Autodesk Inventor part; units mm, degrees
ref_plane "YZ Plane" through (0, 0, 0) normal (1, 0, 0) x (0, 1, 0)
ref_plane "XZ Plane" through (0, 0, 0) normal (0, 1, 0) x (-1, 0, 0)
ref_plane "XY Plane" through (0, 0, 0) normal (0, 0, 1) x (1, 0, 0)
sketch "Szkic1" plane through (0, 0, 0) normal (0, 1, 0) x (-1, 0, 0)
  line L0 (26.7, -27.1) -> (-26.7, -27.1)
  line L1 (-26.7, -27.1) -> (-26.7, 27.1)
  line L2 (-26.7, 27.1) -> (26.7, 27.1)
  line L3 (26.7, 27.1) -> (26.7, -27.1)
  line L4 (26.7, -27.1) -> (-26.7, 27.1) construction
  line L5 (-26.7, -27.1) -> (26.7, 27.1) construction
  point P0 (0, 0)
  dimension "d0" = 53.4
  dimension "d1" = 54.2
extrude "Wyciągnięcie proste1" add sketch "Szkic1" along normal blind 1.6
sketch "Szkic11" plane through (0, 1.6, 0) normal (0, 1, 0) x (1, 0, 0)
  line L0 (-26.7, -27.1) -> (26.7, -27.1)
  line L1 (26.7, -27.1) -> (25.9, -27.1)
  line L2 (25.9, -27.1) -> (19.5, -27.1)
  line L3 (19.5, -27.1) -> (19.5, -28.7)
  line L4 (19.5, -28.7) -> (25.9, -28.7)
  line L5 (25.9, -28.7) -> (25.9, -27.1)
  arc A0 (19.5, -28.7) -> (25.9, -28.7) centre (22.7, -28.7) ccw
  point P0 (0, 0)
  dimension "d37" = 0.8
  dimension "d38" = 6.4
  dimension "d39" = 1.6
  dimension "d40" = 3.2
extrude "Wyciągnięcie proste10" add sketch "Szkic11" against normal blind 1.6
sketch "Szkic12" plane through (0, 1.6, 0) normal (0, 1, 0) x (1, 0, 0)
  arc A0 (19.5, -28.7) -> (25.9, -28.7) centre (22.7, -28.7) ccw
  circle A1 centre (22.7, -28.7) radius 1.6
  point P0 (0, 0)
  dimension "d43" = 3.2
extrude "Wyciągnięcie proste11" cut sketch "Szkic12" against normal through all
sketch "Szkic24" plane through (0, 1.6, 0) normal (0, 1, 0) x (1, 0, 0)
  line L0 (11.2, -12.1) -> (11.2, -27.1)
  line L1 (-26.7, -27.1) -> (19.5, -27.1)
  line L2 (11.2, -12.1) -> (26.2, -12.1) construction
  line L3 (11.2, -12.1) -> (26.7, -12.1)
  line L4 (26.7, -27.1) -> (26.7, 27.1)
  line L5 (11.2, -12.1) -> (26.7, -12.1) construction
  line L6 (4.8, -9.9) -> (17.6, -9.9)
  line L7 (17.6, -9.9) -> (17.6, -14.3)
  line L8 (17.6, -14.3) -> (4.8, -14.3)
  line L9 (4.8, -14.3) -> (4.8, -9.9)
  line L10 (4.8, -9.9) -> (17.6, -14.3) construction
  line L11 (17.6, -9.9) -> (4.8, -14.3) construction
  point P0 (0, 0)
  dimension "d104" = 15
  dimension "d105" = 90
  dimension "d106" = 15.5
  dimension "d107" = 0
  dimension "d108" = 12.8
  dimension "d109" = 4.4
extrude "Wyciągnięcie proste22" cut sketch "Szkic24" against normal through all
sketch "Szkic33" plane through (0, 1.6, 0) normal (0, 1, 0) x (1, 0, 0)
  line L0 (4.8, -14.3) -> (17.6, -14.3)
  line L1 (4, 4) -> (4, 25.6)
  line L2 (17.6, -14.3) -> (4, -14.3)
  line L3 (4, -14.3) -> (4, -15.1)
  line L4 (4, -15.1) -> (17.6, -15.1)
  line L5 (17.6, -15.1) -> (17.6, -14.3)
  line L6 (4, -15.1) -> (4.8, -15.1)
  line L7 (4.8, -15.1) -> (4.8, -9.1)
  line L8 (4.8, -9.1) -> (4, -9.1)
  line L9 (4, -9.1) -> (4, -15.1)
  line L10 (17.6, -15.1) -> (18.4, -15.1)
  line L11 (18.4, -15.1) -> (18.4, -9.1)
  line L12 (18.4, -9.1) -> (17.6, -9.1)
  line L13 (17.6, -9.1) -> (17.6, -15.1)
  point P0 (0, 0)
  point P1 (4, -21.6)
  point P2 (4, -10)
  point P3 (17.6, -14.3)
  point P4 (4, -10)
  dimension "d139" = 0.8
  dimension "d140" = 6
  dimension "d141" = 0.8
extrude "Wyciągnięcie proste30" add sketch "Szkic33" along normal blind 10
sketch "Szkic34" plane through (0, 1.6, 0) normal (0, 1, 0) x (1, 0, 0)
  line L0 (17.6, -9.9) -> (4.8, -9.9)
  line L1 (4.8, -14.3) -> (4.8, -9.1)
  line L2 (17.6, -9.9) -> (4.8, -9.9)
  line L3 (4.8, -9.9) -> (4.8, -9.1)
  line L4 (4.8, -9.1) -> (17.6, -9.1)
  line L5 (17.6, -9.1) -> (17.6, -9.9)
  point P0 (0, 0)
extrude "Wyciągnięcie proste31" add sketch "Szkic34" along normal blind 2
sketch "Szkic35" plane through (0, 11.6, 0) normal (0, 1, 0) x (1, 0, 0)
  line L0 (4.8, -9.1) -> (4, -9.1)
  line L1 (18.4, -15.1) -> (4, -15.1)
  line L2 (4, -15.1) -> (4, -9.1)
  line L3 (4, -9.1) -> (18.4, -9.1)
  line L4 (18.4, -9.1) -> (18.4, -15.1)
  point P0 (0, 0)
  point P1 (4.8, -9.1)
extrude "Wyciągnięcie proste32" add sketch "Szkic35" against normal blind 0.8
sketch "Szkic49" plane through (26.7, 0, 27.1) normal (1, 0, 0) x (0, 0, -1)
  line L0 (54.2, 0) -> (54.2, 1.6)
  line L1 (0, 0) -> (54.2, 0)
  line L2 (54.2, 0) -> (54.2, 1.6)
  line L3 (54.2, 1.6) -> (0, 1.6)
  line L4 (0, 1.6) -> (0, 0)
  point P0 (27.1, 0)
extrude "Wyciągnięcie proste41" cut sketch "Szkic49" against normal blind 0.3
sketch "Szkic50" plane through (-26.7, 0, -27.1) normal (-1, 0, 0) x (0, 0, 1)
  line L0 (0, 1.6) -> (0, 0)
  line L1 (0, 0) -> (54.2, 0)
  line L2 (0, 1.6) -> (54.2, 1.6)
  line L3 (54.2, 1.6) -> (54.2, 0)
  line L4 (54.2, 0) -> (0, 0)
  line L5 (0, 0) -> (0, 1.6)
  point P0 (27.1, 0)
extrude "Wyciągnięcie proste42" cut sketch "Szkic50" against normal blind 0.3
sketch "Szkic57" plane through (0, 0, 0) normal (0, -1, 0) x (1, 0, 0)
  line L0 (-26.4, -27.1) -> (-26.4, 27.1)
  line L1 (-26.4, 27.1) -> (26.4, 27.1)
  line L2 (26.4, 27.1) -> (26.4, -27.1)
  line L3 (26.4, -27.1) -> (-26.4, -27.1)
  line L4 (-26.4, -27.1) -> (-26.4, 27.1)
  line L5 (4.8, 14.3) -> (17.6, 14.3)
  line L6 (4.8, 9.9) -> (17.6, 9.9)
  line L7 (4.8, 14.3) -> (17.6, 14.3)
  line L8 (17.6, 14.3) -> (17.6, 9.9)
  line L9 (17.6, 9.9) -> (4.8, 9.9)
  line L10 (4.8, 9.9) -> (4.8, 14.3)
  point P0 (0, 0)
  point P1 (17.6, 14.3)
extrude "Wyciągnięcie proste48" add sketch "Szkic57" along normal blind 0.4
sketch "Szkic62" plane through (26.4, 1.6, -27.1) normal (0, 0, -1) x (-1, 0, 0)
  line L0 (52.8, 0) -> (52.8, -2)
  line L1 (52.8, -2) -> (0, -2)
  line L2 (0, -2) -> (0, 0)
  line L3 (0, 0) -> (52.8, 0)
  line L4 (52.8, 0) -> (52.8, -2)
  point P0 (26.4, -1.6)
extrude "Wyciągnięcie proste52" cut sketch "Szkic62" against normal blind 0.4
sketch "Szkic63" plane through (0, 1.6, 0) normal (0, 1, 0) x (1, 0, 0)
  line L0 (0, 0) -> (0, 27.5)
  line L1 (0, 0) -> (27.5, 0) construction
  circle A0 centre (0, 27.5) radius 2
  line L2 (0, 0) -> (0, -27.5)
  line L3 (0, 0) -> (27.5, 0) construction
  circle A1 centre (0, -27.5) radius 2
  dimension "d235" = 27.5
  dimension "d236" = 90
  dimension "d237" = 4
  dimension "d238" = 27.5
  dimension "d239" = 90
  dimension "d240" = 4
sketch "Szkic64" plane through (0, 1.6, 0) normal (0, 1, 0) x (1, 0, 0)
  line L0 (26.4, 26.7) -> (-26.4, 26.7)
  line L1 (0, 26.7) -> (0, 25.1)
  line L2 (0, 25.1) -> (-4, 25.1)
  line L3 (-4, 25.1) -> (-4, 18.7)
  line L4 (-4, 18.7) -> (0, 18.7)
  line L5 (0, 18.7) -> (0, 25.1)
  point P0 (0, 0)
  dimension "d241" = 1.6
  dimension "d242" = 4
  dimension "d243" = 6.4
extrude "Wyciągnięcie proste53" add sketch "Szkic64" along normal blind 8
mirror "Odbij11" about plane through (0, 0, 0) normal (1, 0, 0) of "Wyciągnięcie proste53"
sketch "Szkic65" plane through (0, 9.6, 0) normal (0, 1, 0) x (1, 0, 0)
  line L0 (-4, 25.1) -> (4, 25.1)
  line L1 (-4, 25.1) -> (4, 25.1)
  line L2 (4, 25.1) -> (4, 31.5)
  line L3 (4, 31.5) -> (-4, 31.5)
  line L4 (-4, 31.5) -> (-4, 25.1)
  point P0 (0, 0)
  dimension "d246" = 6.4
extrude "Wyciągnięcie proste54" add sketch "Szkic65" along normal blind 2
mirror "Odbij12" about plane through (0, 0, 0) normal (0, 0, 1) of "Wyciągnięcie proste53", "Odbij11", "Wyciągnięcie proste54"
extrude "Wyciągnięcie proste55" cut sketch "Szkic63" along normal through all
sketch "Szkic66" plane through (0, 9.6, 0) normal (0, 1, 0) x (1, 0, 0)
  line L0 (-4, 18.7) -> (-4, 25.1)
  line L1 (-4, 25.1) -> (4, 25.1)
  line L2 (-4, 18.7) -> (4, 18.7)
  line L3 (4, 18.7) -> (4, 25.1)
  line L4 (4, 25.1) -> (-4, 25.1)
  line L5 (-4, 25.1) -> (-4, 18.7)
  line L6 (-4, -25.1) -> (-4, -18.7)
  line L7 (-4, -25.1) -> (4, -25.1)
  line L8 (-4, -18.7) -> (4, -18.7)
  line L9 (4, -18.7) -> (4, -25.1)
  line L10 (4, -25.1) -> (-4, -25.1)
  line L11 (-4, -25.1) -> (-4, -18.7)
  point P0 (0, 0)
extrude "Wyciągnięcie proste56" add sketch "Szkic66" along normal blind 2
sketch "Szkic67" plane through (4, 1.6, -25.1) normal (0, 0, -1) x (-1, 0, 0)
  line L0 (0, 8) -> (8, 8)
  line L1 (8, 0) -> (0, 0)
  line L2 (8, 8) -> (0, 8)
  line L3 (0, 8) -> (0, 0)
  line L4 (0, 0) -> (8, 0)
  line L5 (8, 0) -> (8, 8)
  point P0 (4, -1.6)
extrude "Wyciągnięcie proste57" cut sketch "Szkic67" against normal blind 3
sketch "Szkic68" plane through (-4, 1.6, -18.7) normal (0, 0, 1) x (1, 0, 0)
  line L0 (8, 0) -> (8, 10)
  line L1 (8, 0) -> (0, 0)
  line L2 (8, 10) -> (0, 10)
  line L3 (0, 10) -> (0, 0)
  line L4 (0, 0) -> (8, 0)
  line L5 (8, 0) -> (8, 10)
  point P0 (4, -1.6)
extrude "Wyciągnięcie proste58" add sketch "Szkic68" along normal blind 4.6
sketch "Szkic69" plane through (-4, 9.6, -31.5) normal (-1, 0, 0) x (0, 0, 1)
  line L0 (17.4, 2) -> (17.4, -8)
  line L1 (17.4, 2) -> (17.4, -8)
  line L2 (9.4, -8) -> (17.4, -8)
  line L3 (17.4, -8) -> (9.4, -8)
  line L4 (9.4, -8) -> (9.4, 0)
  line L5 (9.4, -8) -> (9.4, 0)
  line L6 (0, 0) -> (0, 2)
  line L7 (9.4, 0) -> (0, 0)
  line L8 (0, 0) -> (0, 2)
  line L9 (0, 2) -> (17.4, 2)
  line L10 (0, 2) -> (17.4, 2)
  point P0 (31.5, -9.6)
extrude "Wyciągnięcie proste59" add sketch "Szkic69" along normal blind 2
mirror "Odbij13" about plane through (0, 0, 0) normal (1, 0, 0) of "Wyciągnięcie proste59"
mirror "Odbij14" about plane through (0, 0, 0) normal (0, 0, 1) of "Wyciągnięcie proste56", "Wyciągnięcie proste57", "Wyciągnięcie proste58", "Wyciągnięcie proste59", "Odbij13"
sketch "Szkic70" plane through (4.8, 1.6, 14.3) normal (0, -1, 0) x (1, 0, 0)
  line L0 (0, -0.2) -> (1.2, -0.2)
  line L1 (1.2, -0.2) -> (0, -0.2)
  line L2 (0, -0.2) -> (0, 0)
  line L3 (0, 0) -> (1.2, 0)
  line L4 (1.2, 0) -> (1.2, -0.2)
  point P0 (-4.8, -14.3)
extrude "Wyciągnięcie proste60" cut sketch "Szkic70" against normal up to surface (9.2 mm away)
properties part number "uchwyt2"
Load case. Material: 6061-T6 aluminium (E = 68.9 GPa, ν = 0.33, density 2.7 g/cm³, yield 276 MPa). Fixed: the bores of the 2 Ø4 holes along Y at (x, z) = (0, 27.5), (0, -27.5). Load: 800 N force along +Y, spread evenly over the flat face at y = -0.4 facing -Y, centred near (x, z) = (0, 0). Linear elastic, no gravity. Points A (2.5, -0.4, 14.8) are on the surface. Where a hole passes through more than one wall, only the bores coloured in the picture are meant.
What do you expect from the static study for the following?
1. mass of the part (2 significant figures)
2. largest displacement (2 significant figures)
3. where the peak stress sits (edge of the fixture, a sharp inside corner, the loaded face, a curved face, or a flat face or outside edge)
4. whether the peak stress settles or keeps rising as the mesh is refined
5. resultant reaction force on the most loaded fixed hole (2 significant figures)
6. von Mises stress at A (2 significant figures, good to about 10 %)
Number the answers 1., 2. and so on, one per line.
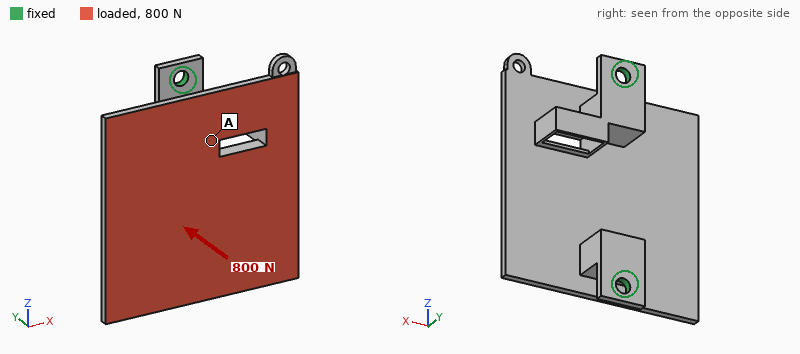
1. 22 g
2. 0.25 mm
3. edge of the fixture
4. keeps rising
5. 540 N
6. 20 MPa
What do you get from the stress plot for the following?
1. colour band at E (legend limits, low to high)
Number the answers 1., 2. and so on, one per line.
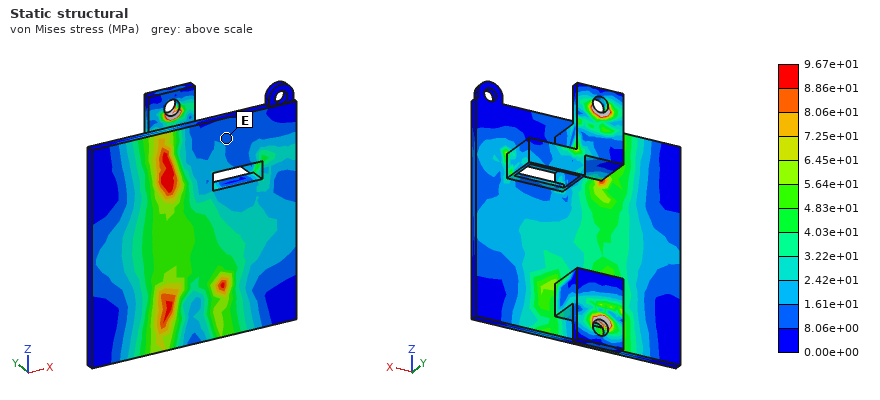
1. 8.06e+00 to 1.61e+01 MPa
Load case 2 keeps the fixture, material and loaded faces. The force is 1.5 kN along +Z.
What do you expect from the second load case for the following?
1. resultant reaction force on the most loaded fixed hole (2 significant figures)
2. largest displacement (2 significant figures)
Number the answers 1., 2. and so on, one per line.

1. 830 N
2. 0.14 mm
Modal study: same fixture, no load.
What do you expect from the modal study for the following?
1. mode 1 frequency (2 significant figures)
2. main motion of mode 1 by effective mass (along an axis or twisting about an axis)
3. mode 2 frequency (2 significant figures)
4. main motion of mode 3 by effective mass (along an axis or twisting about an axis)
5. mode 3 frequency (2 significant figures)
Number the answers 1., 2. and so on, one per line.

1. 1500 Hz
2. along X
3. 3000 Hz
4. along Y
5. 3400 Hz
